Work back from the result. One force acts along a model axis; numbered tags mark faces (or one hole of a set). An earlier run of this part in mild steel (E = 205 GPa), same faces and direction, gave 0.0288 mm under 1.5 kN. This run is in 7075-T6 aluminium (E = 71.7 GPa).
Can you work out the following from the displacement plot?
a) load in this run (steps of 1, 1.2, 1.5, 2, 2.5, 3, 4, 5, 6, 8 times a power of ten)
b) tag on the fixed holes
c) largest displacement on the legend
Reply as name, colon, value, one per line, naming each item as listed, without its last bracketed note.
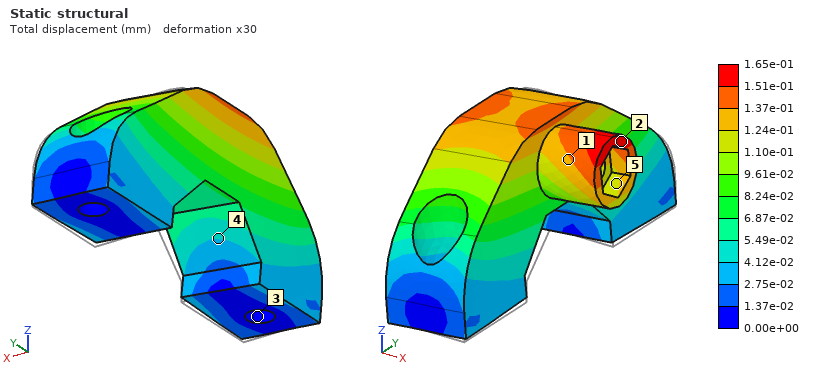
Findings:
load in this run: 3 kN
tag on the fixed holes: 3
largest displacement on the legend: 1.65e-01 mm
